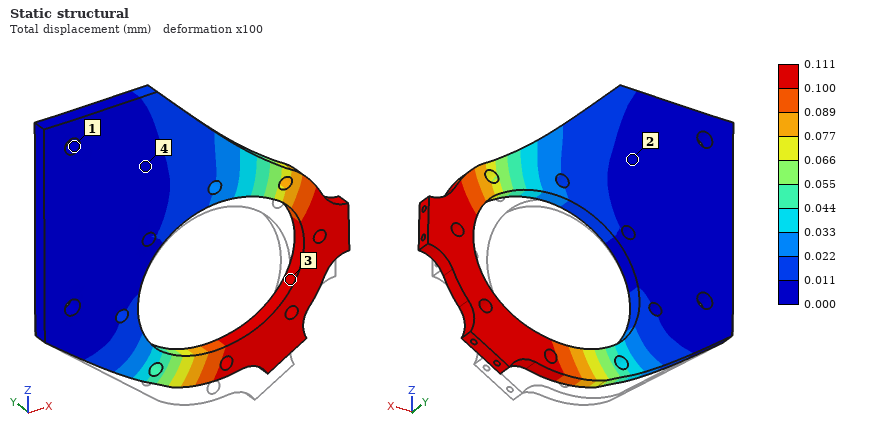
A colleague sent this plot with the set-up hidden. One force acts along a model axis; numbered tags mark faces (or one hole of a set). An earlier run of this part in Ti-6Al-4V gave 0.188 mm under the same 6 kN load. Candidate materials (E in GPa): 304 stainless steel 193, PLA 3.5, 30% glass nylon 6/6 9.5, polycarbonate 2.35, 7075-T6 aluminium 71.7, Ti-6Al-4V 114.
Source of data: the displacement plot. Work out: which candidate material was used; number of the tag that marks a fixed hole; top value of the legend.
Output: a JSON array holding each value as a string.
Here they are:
["304 stainless steel", "1", "0.111 mm"]
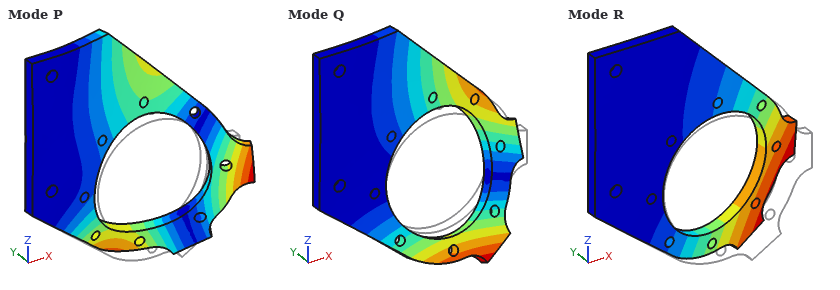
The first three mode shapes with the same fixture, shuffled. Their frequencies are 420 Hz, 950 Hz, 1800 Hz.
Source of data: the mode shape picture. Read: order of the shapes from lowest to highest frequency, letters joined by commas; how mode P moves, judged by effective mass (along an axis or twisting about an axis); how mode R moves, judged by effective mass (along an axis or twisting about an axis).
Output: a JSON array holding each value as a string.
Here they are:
["R, Q, P", "along Y", "along Y"]
